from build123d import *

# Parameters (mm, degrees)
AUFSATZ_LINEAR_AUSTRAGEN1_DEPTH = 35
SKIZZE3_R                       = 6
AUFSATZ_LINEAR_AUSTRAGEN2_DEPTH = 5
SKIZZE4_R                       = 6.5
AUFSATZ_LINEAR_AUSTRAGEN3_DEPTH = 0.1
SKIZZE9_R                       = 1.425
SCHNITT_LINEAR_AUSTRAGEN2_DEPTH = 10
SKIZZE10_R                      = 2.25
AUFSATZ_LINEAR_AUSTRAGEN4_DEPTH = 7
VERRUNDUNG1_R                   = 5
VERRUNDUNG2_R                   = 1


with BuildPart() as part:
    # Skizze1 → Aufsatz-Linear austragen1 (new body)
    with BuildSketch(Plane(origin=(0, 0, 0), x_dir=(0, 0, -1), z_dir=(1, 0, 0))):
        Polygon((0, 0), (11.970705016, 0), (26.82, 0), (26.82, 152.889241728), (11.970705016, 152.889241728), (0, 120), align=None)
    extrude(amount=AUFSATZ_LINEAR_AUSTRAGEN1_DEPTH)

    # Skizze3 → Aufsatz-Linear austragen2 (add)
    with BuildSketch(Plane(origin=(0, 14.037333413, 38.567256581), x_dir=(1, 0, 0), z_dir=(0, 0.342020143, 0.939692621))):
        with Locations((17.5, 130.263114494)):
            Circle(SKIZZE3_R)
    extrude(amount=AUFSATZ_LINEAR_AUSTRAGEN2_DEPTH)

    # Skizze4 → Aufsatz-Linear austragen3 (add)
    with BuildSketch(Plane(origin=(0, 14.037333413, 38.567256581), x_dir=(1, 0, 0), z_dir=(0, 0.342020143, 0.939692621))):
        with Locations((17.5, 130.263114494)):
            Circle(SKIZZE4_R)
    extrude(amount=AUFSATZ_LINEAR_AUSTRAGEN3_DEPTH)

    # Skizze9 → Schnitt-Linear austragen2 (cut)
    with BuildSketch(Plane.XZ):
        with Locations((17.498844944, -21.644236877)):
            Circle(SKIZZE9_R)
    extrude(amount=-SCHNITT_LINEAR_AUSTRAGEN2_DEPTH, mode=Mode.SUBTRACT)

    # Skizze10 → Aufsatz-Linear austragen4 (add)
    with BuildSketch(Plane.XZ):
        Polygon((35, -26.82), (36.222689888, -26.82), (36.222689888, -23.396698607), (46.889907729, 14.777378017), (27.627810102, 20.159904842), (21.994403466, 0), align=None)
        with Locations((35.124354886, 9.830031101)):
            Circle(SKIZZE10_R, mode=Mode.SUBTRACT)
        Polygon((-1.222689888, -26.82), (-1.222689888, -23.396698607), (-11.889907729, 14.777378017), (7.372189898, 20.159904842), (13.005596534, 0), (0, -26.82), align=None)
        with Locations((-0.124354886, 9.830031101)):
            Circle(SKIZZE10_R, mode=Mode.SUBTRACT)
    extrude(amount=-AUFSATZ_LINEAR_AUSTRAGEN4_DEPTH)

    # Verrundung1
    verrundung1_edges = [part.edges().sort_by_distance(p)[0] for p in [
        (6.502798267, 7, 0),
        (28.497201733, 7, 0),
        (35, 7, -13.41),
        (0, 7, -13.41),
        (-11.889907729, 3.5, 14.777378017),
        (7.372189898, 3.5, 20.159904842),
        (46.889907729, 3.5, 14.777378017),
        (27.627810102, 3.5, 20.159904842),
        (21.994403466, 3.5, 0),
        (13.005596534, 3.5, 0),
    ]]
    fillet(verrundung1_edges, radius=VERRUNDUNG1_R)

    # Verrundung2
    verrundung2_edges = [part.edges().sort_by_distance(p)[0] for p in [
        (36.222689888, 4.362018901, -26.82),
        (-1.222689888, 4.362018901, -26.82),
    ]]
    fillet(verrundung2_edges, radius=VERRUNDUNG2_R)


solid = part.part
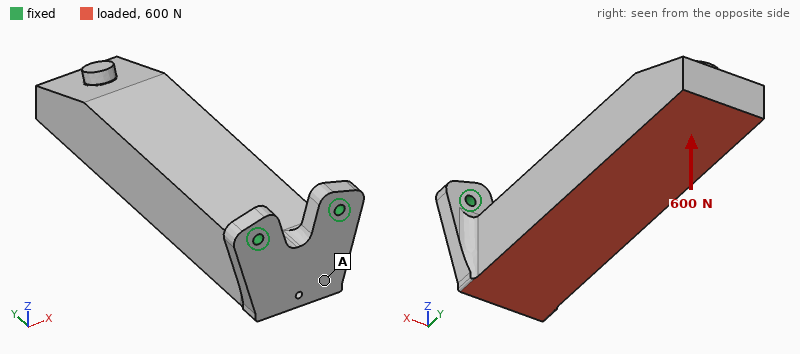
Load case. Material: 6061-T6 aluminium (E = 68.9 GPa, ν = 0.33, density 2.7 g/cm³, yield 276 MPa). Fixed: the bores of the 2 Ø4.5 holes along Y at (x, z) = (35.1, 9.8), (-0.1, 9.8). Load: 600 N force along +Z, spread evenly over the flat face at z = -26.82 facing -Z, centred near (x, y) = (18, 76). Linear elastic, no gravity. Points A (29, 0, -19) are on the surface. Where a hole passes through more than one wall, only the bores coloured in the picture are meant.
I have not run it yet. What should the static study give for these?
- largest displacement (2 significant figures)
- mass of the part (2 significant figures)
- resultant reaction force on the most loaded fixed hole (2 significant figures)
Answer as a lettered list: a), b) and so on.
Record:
a) 1.1 mm
b) 390 g
c) 350 N
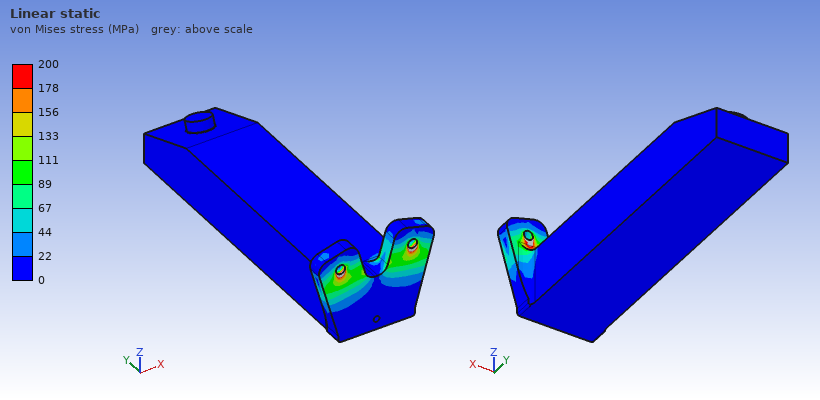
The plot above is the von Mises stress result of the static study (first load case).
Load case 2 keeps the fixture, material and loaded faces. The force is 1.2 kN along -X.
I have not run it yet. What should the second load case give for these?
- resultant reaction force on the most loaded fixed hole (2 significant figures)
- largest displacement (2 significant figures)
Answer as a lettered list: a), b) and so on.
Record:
a) 2.7 kN
b) 0.31 mm
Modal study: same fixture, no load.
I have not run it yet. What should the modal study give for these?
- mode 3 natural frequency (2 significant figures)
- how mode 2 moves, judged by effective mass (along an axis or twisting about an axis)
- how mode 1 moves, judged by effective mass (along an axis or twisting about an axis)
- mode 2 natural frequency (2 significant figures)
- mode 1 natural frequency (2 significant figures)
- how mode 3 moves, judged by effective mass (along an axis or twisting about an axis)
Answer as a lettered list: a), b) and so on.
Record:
a) 2900 Hz
b) along X
c) along Z
d) 660 Hz
e) 240 Hz
f) along Y
